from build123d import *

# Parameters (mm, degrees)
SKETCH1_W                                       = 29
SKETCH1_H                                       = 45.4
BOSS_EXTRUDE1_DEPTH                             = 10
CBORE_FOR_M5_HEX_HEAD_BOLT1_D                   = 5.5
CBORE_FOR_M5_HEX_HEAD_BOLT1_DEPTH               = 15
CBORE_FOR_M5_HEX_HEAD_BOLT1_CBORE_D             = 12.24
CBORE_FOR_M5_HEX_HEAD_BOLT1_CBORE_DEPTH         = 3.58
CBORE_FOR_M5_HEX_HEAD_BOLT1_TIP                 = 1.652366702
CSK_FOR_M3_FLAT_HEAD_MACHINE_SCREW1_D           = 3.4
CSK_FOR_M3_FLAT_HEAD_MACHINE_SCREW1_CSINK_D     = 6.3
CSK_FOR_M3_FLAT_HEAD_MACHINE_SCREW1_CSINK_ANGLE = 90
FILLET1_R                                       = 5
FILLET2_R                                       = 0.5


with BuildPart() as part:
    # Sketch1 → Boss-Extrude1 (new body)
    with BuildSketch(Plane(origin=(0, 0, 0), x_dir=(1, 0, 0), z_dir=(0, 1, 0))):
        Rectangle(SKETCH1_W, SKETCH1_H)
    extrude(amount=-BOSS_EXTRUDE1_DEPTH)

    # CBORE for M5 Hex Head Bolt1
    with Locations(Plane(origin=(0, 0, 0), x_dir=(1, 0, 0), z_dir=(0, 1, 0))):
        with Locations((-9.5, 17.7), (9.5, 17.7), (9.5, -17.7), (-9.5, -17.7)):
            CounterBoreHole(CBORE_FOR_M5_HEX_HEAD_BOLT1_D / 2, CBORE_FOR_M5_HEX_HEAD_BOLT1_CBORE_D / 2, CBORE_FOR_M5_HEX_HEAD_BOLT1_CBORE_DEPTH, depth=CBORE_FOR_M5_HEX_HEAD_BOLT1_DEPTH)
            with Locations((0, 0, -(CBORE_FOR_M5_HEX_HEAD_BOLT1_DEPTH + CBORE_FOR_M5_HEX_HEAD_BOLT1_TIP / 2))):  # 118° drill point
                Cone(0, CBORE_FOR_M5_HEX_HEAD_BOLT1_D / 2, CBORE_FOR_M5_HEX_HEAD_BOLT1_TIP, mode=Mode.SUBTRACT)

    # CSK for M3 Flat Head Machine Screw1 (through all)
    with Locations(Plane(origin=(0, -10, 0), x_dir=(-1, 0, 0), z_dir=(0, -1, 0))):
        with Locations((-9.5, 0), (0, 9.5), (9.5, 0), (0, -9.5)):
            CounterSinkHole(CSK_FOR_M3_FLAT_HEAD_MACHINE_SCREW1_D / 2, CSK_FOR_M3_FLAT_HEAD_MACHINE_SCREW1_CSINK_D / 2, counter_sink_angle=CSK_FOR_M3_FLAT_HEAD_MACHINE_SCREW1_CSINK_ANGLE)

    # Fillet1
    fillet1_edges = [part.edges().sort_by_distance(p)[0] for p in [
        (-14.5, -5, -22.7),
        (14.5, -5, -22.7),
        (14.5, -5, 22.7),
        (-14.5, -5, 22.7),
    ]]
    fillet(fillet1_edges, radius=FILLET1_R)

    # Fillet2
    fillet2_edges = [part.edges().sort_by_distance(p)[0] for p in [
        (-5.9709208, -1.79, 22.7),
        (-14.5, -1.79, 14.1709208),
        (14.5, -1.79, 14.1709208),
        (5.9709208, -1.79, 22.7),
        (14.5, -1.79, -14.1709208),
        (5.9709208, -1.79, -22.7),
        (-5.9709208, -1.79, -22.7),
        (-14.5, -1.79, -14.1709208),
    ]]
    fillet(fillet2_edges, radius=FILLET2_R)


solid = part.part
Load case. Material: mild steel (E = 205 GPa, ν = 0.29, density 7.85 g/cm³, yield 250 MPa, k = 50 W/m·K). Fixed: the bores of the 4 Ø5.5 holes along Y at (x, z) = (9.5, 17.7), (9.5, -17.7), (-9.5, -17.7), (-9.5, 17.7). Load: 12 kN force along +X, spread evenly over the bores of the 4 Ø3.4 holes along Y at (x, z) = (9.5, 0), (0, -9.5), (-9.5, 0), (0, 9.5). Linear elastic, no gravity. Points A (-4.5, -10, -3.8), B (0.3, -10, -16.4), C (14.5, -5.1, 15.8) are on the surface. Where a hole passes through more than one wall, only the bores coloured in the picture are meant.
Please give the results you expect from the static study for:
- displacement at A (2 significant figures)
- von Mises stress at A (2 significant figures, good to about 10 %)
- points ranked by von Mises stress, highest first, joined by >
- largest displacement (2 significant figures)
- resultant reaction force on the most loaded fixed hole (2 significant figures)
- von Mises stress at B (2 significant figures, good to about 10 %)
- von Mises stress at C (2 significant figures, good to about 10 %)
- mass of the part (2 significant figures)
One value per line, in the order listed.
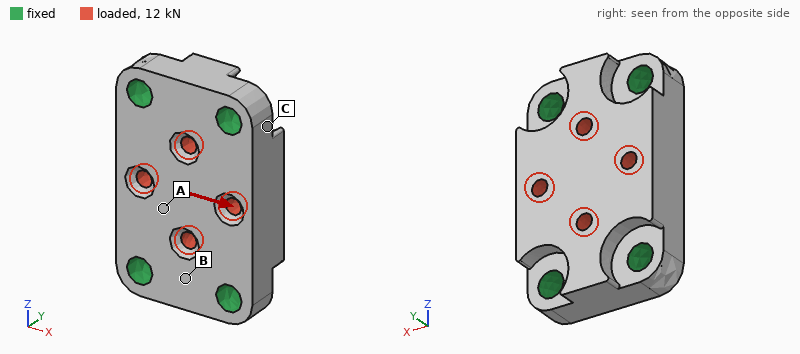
4.1 µm
15 MPa
C > B > A
6.6 µm
3.5 kN
28 MPa
49 MPa
82 g
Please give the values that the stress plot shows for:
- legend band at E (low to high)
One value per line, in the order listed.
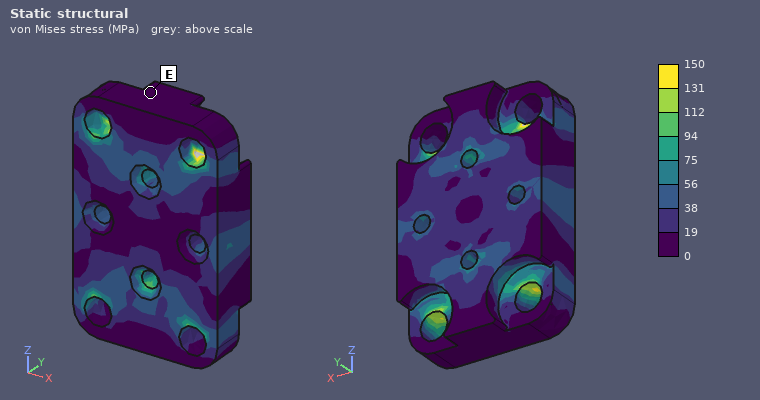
0 to 19 MPa
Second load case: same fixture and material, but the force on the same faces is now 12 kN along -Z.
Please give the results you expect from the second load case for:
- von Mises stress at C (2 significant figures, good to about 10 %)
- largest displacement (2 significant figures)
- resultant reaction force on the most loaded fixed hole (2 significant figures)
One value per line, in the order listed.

21 MPa
2.5 µm
3.1 kN
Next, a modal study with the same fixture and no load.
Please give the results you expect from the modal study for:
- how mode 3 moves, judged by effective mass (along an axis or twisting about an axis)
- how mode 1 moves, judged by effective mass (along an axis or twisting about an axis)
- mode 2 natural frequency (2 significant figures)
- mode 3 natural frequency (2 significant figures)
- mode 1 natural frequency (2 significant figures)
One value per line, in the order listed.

along X
along Y
32 kHz
37 kHz
26 kHz
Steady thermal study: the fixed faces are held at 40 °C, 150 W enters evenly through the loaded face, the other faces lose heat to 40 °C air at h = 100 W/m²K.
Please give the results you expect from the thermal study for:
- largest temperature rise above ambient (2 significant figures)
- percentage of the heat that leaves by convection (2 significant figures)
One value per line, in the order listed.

83 K
9.2 %
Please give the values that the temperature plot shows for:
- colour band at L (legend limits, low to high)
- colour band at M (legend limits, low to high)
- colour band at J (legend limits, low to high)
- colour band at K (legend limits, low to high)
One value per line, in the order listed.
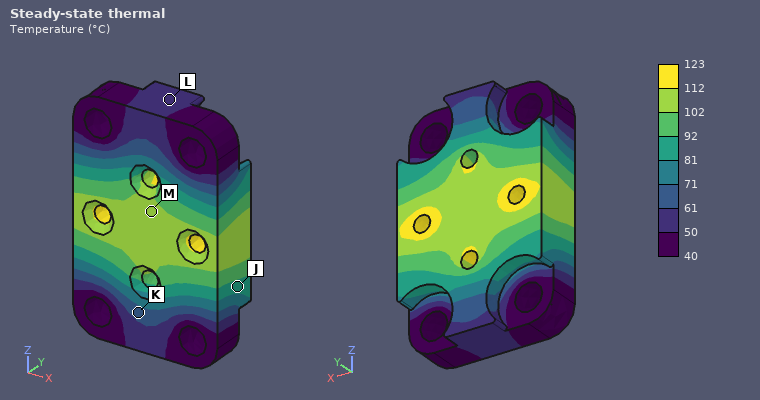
50 to 61 °C
102 to 112 °C
81 to 92 °C
61 to 71 °C
